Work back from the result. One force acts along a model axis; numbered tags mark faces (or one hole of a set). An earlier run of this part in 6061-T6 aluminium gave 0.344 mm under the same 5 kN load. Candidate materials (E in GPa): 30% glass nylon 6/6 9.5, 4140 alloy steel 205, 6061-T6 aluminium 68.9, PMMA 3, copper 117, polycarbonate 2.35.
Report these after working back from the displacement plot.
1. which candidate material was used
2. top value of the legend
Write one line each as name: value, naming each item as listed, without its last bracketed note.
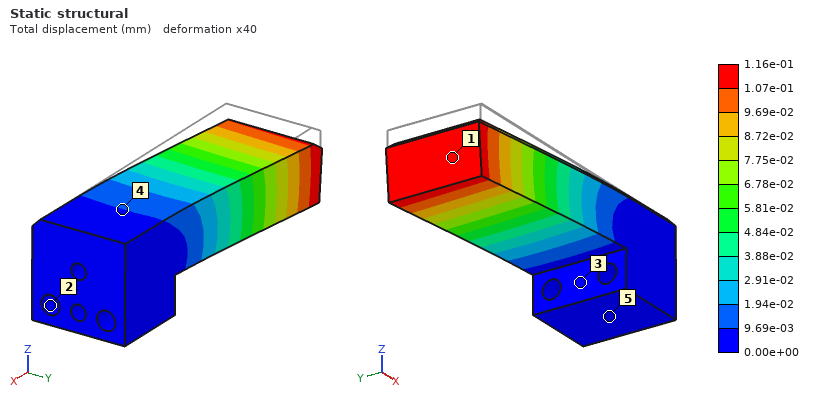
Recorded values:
which candidate material was used: 4140 alloy steel
top value of the legend: 1.16e-01 mm
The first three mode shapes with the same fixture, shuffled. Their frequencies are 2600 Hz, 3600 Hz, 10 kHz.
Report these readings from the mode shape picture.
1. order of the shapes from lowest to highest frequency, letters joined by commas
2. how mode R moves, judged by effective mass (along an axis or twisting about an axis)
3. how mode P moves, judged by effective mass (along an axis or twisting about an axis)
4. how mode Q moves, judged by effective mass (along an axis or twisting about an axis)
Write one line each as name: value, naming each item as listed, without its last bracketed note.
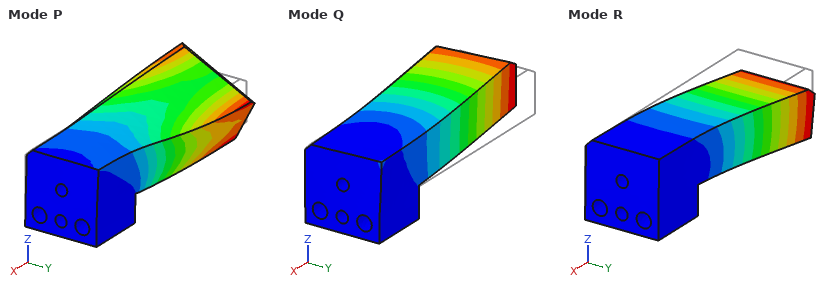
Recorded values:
order of the shapes from lowest to highest frequency, letters joined by commas: R, Q, P
how mode R moves, judged by effective mass: along Z
how mode P moves, judged by effective mass: twisting about X
how mode Q moves, judged by effective mass: along Y
